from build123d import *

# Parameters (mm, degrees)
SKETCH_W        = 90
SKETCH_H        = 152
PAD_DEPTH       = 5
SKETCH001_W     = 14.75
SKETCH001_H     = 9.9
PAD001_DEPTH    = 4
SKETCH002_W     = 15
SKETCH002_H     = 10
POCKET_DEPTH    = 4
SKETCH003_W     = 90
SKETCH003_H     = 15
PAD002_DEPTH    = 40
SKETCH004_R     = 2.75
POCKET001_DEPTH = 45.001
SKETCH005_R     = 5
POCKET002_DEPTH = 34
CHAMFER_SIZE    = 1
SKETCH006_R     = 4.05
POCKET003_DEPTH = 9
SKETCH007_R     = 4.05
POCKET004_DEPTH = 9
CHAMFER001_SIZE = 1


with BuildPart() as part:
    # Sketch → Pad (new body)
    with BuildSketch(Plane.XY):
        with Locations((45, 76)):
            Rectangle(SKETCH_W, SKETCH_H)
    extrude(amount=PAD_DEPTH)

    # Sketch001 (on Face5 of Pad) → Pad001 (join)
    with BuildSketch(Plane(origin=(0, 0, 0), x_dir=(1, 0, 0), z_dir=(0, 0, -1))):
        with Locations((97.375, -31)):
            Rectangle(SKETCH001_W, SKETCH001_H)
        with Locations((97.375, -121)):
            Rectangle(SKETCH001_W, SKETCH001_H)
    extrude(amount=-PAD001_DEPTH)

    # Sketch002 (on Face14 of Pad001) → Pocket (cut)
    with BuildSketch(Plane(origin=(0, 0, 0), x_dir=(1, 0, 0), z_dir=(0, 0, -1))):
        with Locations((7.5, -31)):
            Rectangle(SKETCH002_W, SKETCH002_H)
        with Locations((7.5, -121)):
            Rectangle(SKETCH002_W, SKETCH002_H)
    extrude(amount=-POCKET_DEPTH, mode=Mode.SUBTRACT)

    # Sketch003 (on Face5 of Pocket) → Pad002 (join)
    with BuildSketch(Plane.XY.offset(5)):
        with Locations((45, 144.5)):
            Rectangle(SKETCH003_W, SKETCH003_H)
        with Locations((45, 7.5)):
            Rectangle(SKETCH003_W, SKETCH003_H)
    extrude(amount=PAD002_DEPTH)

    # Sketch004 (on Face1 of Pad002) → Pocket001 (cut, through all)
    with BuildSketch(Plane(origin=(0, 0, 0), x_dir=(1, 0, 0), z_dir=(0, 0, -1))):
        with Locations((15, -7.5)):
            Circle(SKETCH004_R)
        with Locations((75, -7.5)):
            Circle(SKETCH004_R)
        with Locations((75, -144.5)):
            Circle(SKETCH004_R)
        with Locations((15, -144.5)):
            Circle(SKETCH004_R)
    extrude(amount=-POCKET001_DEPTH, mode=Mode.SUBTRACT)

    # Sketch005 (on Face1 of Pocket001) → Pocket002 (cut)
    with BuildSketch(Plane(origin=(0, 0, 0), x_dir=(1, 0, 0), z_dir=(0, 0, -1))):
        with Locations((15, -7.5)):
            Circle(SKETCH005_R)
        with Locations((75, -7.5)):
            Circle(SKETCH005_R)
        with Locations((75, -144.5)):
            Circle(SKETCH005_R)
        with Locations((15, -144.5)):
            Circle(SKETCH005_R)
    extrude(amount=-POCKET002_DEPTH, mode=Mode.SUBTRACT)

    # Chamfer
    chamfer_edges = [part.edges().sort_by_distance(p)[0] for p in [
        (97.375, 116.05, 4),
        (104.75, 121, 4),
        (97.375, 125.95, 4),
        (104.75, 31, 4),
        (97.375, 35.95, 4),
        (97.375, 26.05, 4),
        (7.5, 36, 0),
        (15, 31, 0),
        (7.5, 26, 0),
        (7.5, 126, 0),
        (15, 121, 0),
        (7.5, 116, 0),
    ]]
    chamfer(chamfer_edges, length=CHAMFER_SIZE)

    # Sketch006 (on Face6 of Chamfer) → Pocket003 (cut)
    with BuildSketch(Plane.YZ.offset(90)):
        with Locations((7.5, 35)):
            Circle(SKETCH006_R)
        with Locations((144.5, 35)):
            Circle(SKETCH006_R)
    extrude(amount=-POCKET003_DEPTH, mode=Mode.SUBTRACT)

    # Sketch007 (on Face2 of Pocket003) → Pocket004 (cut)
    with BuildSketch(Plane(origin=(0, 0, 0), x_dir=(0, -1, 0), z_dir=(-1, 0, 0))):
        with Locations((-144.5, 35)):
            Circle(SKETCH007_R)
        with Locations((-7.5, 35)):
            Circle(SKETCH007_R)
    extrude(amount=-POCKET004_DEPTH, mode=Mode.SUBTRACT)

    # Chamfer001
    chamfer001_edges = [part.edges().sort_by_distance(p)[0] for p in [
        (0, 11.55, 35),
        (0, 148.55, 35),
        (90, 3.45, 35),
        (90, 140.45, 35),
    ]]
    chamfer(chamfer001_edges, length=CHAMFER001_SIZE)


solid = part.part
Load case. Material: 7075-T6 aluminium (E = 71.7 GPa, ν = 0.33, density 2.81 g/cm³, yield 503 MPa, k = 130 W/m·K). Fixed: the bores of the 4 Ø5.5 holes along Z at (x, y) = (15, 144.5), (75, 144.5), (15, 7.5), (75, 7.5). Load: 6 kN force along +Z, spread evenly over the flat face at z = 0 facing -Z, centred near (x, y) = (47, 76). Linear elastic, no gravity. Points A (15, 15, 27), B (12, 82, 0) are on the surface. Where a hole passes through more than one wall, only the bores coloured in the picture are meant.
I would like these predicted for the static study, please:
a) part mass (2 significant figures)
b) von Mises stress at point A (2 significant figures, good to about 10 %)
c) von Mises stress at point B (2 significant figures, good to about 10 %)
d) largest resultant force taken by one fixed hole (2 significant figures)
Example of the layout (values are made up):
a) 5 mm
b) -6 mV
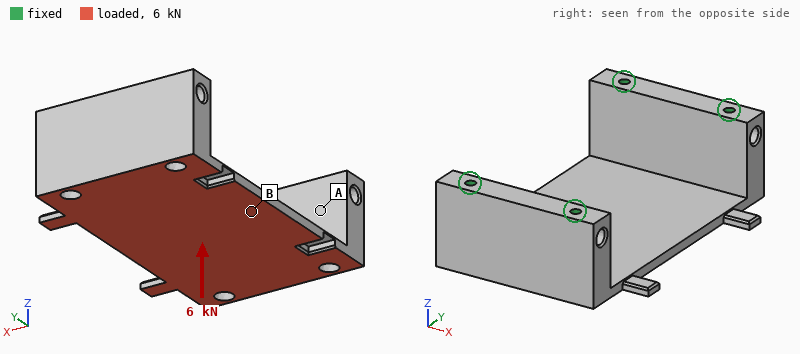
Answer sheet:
a) 460 g
b) 14 MPa
c) 76 MPa
d) 1.9 kN
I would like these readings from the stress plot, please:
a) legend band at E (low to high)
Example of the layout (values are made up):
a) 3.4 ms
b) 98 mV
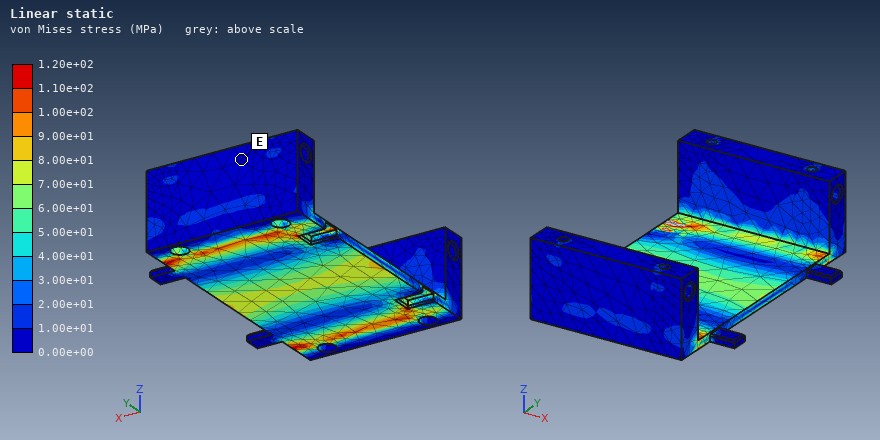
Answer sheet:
a) 0.00e+00 to 1.00e+01 MPa
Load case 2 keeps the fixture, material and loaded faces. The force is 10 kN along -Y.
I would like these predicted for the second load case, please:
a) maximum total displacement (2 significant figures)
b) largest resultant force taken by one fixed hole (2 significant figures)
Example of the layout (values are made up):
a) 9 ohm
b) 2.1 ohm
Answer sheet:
a) 0.18 mm
b) 2.5 kN
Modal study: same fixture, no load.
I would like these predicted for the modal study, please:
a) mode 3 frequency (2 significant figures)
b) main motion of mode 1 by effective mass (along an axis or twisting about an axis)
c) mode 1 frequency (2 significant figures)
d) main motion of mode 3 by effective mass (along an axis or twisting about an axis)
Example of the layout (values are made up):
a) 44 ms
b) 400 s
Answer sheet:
a) 2500 Hz
b) along Z
c) 1500 Hz
d) along Y
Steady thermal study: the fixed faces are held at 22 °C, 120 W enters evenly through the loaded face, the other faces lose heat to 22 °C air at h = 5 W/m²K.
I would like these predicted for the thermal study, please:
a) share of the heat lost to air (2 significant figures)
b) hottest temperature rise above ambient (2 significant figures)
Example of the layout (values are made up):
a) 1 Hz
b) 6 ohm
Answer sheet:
a) 3.3 %
b) 50 K
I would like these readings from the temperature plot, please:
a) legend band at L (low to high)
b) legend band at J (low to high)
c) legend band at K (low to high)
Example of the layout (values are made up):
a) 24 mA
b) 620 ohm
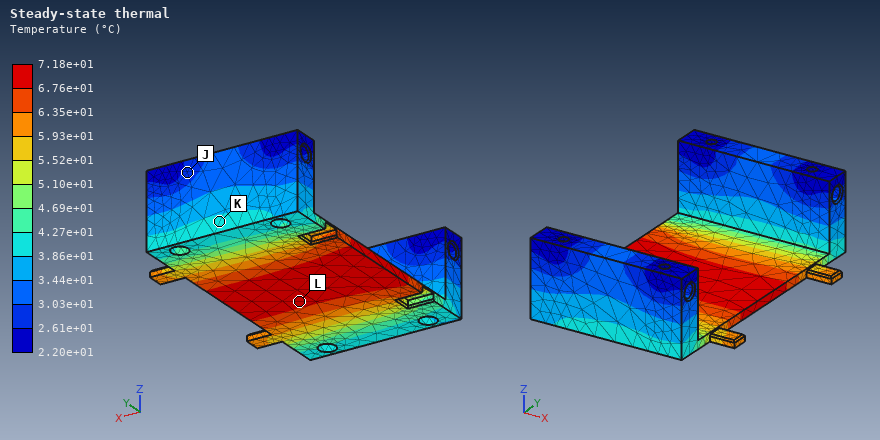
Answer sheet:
a) 6.76e+01 to 7.18e+01 °C
b) 2.61e+01 to 3.03e+01 °C
c) 3.86e+01 to 4.27e+01 °C
